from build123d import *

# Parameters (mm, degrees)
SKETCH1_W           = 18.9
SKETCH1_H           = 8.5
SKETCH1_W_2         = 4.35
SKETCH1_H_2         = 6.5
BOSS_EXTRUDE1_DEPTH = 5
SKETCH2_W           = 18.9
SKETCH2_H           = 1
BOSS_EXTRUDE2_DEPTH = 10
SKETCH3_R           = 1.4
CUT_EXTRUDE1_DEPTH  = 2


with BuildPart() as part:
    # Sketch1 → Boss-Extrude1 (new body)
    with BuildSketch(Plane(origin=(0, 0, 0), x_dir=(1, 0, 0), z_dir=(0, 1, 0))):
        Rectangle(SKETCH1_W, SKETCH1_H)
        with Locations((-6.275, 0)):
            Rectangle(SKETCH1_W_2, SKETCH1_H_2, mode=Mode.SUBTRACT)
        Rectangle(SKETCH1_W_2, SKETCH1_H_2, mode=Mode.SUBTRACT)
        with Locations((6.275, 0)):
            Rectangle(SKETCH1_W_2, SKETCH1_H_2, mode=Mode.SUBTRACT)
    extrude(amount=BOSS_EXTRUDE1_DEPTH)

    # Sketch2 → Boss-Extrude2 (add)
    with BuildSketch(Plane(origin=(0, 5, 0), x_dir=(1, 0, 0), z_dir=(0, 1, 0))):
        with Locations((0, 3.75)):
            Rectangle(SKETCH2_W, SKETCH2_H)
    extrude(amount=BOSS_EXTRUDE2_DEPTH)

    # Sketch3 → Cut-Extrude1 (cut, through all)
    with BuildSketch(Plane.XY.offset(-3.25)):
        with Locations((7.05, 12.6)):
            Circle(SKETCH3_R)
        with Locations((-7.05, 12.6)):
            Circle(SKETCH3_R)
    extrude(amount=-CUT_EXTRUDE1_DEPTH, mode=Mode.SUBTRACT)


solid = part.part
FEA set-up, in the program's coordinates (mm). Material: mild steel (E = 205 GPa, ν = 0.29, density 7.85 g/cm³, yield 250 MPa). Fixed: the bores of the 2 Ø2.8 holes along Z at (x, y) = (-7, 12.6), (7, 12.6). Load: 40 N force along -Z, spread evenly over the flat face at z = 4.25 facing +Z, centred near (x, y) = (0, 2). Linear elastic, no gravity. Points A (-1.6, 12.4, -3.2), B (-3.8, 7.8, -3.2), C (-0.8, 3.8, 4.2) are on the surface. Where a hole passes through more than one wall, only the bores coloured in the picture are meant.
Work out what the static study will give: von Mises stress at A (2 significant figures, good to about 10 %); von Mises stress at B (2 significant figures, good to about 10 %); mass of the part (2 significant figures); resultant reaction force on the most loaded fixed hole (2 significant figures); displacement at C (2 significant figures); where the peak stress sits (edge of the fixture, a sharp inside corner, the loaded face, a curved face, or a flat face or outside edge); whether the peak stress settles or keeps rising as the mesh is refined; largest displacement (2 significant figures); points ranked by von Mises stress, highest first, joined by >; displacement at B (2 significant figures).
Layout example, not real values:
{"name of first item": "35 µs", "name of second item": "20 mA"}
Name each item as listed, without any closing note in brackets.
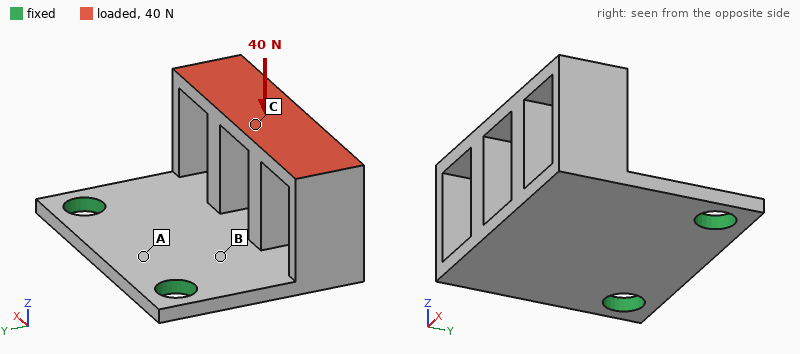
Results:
{"von Mises stress at A": "34 MPa", "von Mises stress at B": "60 MPa", "mass of the part": "4.4 g", "resultant reaction force on the most loaded fixed hole": "20 N", "displacement at C": "52 µm", "where the peak stress sits": "edge of the fixture", "whether the peak stress settles or keeps rising as the mesh is refined": "keeps rising", "largest displacement": "65 µm", "points ranked by von Mises stress, highest first, joined by >": "B > A > C", "displacement at B": "10 µm"}
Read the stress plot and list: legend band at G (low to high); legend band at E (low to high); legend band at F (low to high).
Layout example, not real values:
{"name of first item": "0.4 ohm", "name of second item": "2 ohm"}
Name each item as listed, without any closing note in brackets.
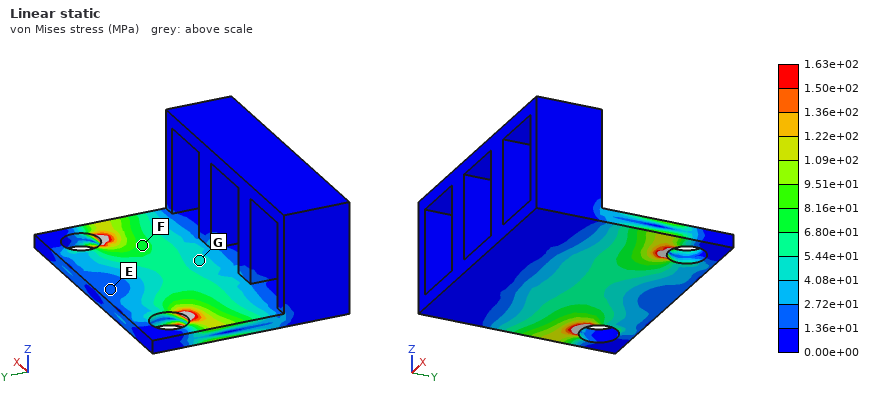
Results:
{"legend band at G": "4.08e+01 to 5.44e+01 MPa", "legend band at E": "1.36e+01 to 2.72e+01 MPa", "legend band at F": "6.80e+01 to 8.16e+01 MPa"}
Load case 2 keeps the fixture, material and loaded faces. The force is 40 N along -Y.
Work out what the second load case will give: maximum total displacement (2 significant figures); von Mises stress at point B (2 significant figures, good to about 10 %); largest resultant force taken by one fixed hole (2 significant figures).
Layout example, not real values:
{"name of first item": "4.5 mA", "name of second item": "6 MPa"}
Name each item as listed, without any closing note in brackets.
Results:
{"maximum total displacement": "87 µm", "von Mises stress at point B": "92 MPa", "largest resultant force taken by one fixed hole": "21 N"}
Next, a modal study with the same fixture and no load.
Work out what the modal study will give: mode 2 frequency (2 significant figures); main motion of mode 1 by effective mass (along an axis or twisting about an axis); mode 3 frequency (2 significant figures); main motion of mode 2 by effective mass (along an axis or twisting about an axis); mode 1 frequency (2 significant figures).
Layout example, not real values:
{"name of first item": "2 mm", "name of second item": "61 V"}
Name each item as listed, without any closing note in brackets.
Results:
{"mode 2 frequency": "6100 Hz", "main motion of mode 1 by effective mass": "along Z", "mode 3 frequency": "11 kHz", "main motion of mode 2 by effective mass": "along X", "mode 1 frequency": "2400 Hz"}
